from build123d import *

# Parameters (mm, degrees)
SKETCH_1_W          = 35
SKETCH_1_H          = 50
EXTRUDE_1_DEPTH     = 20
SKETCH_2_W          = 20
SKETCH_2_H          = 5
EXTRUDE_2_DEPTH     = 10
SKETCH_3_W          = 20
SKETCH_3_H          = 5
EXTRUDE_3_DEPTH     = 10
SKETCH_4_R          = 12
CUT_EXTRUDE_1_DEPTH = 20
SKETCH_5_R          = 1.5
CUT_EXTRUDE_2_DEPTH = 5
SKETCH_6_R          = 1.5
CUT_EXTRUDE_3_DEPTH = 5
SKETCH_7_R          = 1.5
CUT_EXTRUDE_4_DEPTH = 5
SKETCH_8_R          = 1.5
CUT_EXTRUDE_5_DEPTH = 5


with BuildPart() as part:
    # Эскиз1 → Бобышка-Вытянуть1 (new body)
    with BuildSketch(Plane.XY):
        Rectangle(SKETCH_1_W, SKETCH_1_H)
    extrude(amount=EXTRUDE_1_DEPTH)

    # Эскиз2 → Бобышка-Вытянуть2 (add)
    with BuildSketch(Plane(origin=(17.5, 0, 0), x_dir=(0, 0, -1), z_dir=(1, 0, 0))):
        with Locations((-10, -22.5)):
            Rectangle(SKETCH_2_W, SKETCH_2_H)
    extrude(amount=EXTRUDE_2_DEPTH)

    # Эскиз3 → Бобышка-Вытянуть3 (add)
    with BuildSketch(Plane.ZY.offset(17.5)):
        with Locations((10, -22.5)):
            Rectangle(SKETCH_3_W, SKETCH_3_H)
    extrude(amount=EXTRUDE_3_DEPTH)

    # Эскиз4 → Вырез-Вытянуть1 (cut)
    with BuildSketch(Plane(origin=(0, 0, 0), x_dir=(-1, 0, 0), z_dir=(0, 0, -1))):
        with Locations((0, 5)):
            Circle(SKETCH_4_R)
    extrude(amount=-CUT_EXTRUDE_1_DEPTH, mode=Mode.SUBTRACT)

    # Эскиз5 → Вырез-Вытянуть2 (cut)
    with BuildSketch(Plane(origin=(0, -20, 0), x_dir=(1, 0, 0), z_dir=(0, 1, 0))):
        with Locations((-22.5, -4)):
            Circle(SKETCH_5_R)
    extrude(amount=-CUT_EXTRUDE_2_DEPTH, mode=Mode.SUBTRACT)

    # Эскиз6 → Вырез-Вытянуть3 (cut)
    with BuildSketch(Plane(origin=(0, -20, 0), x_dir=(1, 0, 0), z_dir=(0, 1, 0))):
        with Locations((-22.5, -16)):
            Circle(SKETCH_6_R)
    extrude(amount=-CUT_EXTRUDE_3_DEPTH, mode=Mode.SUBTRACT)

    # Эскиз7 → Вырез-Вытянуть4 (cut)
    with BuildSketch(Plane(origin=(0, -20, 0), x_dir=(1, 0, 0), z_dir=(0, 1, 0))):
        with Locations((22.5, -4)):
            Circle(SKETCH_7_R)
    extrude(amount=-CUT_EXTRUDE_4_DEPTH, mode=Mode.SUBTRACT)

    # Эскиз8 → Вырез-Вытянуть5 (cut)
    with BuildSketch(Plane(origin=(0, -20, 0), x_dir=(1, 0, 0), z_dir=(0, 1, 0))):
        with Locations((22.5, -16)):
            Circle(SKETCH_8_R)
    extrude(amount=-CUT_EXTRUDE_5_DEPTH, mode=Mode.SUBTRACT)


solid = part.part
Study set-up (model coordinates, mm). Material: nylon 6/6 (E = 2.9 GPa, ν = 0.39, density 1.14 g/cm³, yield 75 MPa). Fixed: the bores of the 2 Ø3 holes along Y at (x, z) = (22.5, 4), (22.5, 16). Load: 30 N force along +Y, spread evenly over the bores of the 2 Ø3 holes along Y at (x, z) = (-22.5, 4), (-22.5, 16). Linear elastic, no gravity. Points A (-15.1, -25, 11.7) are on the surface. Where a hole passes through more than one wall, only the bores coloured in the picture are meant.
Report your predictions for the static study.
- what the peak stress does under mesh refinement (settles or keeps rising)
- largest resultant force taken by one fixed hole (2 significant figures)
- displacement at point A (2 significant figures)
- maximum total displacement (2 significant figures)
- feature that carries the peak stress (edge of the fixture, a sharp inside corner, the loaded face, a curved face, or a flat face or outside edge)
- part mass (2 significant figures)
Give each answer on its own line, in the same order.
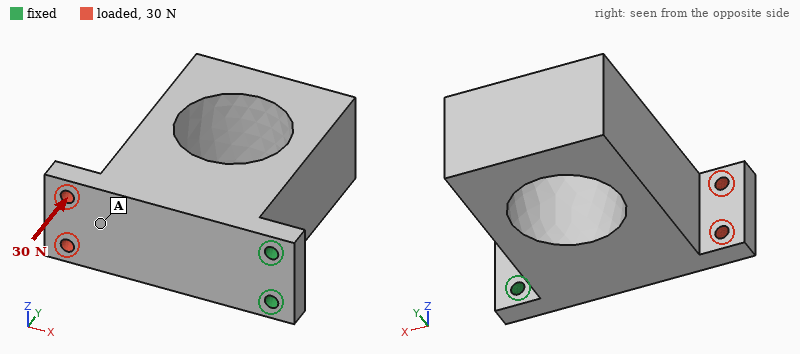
keeps rising
15 N
0.51 mm
0.89 mm
edge of the fixture
32 g
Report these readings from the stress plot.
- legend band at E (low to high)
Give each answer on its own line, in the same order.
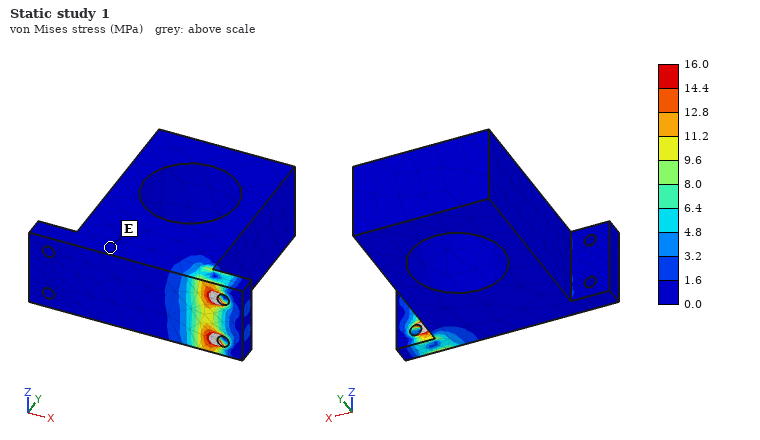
0.0 to 1.6 MPa
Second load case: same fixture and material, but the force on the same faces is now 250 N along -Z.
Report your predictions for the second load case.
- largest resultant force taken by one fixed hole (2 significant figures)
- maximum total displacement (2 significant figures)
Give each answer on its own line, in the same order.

840 N
0.81 mm
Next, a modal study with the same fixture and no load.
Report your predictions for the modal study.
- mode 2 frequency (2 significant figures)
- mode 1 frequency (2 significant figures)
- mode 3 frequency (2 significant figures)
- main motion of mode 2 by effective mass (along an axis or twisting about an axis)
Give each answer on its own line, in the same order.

580 Hz
240 Hz
1300 Hz
along Z
